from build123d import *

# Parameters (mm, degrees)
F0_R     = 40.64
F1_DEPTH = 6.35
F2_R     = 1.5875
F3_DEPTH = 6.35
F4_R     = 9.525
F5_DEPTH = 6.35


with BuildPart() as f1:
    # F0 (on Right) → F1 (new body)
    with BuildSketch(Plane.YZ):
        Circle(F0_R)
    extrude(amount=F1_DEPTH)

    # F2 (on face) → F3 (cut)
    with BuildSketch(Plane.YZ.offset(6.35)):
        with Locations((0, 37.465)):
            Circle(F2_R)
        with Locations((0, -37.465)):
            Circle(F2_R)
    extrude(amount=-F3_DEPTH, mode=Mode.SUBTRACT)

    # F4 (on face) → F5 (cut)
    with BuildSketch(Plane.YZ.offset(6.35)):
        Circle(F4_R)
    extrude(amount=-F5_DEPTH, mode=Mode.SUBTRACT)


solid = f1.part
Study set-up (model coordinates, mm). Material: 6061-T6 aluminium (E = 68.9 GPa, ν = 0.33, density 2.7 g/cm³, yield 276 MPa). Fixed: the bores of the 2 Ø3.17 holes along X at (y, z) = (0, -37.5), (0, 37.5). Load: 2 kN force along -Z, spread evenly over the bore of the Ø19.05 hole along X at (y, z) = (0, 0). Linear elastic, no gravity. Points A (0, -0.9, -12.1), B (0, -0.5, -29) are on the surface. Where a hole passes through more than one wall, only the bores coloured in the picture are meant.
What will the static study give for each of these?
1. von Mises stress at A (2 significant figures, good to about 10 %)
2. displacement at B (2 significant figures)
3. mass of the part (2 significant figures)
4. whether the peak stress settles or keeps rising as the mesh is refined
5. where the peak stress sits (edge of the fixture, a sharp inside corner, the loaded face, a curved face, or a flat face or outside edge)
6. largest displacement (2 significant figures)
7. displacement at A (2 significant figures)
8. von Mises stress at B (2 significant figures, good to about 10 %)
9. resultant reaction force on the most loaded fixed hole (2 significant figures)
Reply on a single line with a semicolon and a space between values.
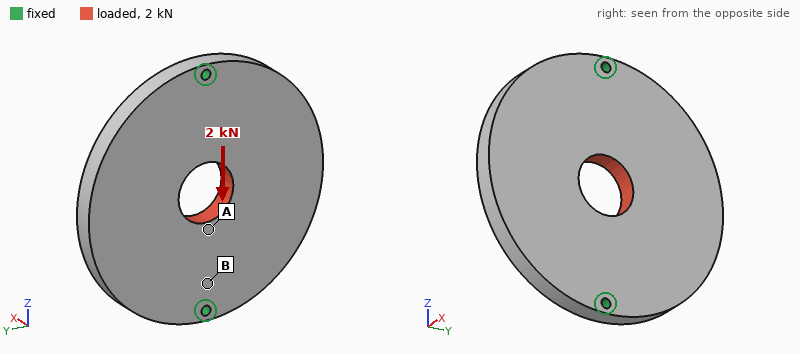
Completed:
5.9 MPa; 1.6 µm; 84 g; keeps rising; edge of the fixture; 4.2 µm; 3.4 µm; 11 MPa; 1.0 kN
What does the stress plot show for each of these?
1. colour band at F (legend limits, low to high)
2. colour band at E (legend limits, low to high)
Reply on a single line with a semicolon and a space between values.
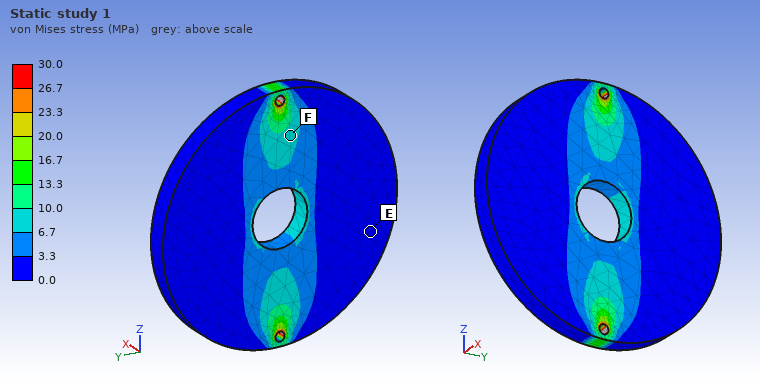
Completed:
6.7 to 10.0 MPa; 0.0 to 3.3 MPa
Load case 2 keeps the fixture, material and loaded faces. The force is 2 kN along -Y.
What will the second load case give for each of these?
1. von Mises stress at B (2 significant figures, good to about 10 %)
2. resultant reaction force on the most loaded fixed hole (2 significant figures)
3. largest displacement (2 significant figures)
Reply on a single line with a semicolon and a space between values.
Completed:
4.8 MPa; 1.0 kN; 5.9 µm
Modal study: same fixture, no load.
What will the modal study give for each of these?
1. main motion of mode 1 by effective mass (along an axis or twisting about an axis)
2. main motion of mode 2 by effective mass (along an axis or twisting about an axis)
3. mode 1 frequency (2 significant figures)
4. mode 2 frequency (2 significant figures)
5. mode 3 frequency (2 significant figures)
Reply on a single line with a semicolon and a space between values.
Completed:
twisting about Z; along X; 2000 Hz; 2800 Hz; 6500 Hz
